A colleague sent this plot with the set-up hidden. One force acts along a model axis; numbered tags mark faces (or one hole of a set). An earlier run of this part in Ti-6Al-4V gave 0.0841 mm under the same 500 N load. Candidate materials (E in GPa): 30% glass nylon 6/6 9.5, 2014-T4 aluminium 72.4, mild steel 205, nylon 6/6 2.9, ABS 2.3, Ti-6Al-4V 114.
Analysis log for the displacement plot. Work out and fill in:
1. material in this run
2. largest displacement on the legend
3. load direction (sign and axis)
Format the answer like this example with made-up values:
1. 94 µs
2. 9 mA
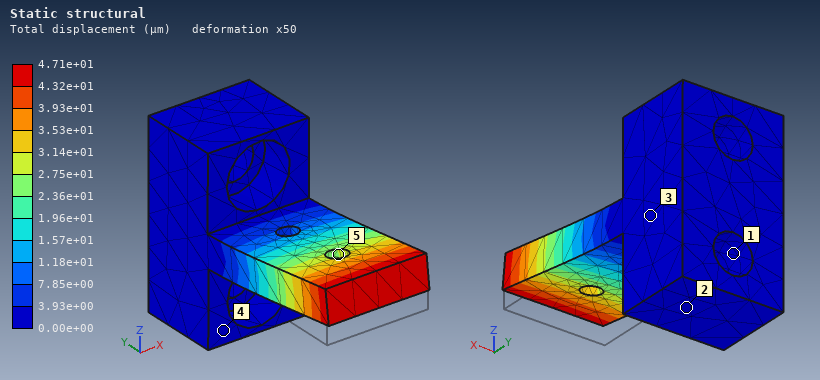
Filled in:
1. mild steel
2. 4.71e+01 µm
3. +Z
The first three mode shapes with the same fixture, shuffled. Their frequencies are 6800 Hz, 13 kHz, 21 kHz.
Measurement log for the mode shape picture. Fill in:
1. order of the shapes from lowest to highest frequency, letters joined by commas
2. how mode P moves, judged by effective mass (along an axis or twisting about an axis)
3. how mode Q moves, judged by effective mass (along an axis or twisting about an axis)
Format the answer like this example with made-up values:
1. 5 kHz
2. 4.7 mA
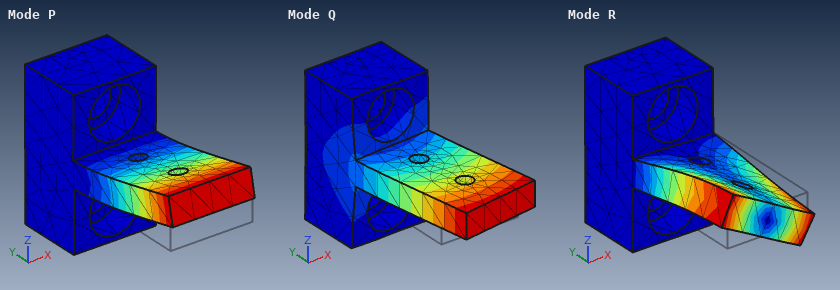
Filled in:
1. P, Q, R
2. along Z
3. along X
